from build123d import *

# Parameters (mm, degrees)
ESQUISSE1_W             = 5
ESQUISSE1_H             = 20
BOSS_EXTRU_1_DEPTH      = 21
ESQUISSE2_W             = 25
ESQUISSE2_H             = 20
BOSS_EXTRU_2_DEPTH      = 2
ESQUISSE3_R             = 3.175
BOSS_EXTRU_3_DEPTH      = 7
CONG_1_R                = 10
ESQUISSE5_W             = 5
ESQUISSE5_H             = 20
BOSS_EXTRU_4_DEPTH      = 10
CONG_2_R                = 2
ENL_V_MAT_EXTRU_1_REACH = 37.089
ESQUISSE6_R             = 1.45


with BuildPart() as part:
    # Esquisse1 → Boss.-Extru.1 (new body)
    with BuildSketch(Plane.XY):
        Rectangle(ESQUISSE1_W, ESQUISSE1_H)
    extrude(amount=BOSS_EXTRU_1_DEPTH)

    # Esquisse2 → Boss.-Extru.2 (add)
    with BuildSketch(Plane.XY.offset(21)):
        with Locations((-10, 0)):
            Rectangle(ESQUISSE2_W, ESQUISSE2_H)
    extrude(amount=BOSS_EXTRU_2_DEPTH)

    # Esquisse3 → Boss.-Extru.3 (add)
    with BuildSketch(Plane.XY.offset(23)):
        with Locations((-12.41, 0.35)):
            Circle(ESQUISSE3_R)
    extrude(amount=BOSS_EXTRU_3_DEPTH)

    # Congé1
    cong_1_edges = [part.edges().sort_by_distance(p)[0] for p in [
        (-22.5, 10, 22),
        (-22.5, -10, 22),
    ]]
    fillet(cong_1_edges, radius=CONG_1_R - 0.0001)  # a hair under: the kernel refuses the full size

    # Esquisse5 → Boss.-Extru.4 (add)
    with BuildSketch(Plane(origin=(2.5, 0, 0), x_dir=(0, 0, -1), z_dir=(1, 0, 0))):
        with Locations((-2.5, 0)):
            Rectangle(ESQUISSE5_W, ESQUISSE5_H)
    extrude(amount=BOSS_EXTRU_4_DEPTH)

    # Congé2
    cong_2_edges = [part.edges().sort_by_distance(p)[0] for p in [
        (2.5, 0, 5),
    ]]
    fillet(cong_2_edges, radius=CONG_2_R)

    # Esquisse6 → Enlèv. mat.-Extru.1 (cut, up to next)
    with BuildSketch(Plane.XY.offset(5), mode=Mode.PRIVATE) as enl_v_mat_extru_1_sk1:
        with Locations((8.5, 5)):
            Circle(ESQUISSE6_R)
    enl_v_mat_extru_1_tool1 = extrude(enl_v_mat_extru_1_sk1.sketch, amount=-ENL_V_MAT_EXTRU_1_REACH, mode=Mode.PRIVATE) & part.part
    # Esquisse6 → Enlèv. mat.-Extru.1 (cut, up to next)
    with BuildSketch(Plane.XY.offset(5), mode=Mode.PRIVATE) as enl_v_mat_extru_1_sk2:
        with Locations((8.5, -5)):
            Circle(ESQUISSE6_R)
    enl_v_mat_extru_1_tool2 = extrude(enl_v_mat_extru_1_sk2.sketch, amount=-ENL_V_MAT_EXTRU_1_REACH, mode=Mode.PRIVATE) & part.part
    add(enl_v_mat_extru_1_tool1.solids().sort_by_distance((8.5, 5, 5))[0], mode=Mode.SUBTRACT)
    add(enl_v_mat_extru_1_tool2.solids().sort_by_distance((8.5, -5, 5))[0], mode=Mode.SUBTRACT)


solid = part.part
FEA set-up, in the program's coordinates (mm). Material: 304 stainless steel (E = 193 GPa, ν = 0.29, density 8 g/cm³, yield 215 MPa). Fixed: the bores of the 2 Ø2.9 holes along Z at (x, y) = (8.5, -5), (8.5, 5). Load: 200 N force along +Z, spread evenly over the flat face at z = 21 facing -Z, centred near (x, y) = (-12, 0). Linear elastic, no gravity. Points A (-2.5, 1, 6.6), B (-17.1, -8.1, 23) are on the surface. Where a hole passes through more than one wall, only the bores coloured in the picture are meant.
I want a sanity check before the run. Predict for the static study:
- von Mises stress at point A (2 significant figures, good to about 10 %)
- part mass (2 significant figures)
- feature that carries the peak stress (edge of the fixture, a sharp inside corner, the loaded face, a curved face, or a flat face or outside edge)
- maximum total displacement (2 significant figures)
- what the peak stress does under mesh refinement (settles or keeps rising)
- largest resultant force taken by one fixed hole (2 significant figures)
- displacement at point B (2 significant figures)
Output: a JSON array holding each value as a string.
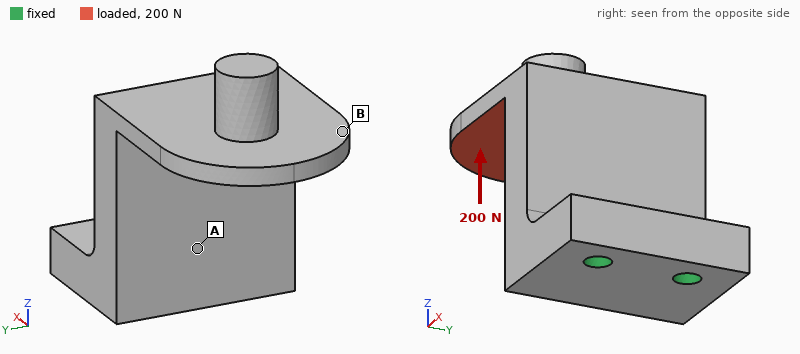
["26 MPa", "33 g", "edge of the fixture", "0.12 mm", "keeps rising", "100 N", "0.083 mm"]
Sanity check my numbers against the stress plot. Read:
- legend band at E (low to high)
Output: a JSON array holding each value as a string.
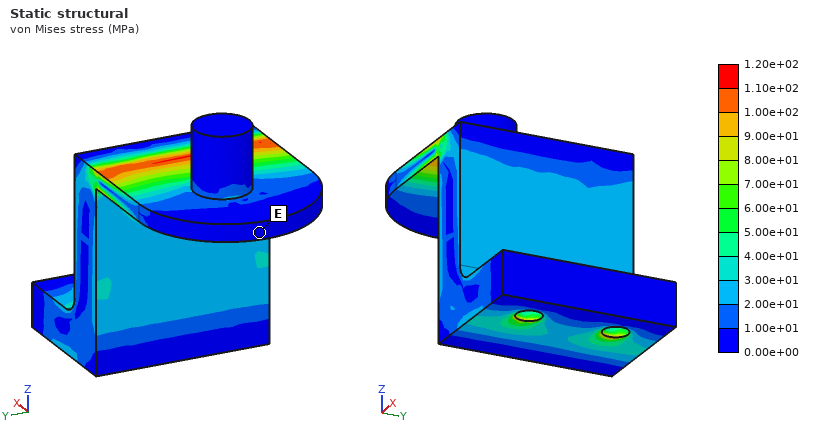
["0.00e+00 to 1.00e+01 MPa"]
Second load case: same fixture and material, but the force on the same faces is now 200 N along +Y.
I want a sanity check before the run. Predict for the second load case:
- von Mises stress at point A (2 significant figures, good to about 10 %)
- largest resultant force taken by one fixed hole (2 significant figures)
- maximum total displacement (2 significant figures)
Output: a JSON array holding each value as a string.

["15 MPa", "430 N", "20 µm"]
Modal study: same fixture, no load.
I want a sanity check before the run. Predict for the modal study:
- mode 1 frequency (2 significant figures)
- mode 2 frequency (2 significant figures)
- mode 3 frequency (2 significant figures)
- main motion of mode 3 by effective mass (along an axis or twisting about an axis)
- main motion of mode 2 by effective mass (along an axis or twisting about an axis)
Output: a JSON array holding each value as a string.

["2700 Hz", "5700 Hz", "6300 Hz", "along Y", "along X"]
